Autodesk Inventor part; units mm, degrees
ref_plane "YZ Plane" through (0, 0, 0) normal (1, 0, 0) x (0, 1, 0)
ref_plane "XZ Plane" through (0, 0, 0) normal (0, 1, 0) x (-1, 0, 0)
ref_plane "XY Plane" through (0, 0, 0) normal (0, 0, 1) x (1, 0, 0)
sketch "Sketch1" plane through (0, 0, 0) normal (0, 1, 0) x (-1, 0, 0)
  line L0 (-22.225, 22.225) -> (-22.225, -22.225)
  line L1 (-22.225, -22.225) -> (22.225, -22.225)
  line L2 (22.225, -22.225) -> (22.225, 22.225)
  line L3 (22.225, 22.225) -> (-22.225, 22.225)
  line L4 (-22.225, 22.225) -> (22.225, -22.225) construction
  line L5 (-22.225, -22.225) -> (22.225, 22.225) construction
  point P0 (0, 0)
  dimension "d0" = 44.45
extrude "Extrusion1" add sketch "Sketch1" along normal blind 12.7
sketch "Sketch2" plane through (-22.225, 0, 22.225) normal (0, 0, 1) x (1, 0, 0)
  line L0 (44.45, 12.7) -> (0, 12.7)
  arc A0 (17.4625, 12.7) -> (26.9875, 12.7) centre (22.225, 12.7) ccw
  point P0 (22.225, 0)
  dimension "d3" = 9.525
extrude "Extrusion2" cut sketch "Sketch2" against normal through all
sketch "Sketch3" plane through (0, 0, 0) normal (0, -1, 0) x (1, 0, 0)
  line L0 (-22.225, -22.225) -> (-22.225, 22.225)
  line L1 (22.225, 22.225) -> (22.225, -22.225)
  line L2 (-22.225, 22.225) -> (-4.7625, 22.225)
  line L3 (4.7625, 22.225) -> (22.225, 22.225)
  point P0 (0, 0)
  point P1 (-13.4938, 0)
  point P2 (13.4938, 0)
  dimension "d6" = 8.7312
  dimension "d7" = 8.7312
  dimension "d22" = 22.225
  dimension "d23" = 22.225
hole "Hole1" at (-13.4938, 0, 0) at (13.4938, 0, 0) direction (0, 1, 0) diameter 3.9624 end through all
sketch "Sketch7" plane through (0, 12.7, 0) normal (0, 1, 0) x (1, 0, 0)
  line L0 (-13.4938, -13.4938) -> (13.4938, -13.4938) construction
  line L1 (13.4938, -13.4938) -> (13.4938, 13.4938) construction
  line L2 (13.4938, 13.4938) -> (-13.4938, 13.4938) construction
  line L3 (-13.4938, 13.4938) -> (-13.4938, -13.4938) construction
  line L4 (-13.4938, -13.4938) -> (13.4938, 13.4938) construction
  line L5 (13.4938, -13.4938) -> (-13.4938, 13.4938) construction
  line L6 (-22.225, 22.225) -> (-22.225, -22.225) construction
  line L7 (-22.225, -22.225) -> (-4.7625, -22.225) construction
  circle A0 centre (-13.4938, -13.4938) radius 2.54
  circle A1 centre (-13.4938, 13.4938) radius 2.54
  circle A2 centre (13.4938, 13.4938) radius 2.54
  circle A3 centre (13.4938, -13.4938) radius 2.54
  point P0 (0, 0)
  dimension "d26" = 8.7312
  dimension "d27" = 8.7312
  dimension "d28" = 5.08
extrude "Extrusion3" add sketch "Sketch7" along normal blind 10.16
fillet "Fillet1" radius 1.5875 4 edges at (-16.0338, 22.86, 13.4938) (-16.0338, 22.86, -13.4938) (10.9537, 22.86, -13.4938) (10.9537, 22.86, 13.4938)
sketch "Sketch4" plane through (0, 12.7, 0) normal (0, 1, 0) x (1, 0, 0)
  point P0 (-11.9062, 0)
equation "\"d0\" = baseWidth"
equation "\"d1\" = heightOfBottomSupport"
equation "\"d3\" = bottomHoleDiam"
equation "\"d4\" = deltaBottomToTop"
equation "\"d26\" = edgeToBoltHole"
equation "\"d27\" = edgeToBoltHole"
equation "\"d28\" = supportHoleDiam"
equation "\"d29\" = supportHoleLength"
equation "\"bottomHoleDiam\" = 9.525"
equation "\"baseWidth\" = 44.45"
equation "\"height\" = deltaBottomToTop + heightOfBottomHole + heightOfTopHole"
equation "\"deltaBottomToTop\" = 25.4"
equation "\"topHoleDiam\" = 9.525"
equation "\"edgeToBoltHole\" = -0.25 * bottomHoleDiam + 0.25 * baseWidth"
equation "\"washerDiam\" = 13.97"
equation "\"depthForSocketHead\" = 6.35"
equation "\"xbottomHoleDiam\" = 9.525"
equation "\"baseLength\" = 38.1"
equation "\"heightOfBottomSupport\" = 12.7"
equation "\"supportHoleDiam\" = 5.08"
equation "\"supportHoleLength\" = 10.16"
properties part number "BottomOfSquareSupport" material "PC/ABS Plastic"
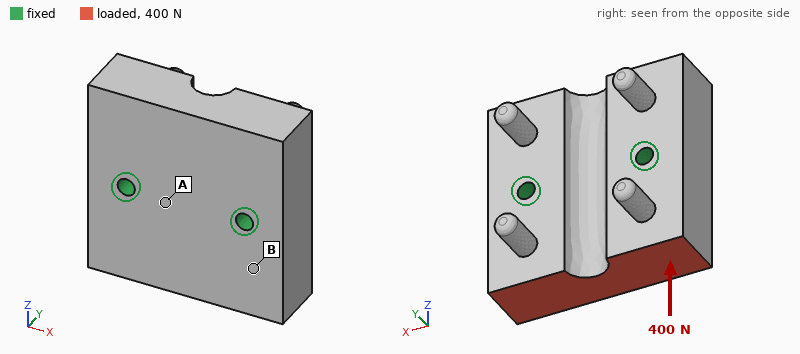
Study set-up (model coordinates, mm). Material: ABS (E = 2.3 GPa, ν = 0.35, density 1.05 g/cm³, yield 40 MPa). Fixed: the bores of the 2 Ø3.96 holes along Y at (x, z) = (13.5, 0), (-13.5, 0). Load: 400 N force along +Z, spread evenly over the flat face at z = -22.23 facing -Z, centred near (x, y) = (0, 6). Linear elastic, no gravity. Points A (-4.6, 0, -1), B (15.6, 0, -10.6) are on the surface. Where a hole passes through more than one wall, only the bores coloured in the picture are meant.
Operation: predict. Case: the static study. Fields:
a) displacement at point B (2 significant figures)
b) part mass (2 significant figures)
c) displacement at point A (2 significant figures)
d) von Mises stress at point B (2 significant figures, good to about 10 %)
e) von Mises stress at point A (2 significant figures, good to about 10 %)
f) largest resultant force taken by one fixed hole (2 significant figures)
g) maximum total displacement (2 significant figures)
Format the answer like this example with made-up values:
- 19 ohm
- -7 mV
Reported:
- 5.3 µm
- 25 g
- 3.8 µm
- 0.91 MPa
- 0.34 MPa
- 200 N
- 9.6 µm
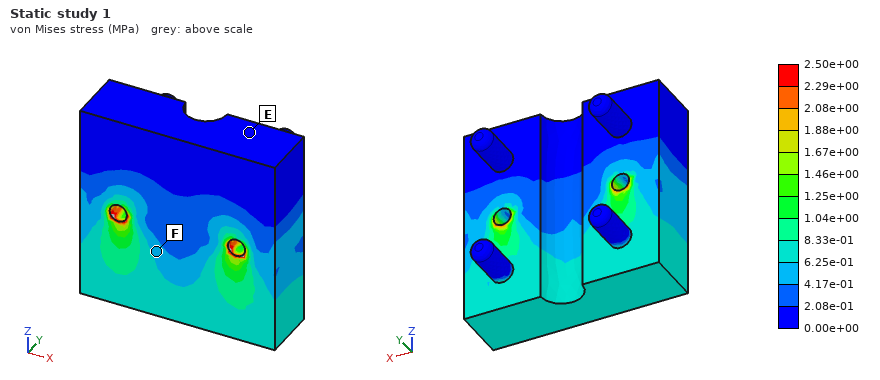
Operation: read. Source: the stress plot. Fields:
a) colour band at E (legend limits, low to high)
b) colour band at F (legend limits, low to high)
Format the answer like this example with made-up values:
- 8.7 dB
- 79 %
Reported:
- 0.00e+00 to 2.08e-01 MPa
- 4.17e-01 to 6.25e-01 MPa
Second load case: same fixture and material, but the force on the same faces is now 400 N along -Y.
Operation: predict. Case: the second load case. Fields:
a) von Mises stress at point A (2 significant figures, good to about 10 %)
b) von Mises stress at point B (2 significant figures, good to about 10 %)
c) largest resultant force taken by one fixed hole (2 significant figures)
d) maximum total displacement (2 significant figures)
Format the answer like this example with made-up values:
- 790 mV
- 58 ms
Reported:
- 3.3 MPa
- 4.5 MPa
- 200 N
- 0.16 mm
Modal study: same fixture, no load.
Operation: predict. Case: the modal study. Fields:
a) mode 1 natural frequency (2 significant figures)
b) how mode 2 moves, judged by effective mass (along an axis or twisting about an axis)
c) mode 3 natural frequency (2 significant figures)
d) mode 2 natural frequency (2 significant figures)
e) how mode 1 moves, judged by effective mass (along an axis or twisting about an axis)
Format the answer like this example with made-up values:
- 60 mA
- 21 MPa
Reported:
- 3700 Hz
- along Y
- 5300 Hz
- 4900 Hz
- twisting about X
